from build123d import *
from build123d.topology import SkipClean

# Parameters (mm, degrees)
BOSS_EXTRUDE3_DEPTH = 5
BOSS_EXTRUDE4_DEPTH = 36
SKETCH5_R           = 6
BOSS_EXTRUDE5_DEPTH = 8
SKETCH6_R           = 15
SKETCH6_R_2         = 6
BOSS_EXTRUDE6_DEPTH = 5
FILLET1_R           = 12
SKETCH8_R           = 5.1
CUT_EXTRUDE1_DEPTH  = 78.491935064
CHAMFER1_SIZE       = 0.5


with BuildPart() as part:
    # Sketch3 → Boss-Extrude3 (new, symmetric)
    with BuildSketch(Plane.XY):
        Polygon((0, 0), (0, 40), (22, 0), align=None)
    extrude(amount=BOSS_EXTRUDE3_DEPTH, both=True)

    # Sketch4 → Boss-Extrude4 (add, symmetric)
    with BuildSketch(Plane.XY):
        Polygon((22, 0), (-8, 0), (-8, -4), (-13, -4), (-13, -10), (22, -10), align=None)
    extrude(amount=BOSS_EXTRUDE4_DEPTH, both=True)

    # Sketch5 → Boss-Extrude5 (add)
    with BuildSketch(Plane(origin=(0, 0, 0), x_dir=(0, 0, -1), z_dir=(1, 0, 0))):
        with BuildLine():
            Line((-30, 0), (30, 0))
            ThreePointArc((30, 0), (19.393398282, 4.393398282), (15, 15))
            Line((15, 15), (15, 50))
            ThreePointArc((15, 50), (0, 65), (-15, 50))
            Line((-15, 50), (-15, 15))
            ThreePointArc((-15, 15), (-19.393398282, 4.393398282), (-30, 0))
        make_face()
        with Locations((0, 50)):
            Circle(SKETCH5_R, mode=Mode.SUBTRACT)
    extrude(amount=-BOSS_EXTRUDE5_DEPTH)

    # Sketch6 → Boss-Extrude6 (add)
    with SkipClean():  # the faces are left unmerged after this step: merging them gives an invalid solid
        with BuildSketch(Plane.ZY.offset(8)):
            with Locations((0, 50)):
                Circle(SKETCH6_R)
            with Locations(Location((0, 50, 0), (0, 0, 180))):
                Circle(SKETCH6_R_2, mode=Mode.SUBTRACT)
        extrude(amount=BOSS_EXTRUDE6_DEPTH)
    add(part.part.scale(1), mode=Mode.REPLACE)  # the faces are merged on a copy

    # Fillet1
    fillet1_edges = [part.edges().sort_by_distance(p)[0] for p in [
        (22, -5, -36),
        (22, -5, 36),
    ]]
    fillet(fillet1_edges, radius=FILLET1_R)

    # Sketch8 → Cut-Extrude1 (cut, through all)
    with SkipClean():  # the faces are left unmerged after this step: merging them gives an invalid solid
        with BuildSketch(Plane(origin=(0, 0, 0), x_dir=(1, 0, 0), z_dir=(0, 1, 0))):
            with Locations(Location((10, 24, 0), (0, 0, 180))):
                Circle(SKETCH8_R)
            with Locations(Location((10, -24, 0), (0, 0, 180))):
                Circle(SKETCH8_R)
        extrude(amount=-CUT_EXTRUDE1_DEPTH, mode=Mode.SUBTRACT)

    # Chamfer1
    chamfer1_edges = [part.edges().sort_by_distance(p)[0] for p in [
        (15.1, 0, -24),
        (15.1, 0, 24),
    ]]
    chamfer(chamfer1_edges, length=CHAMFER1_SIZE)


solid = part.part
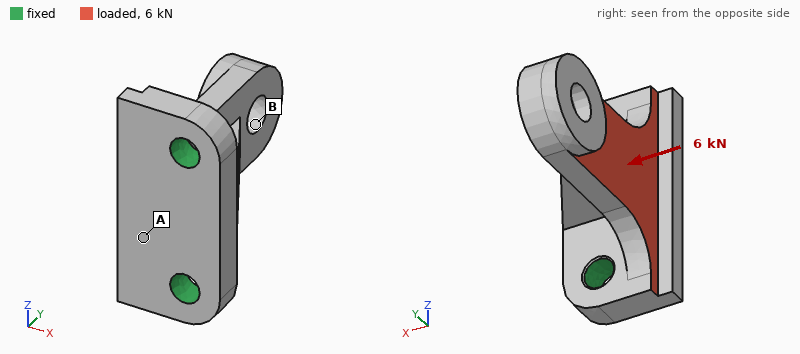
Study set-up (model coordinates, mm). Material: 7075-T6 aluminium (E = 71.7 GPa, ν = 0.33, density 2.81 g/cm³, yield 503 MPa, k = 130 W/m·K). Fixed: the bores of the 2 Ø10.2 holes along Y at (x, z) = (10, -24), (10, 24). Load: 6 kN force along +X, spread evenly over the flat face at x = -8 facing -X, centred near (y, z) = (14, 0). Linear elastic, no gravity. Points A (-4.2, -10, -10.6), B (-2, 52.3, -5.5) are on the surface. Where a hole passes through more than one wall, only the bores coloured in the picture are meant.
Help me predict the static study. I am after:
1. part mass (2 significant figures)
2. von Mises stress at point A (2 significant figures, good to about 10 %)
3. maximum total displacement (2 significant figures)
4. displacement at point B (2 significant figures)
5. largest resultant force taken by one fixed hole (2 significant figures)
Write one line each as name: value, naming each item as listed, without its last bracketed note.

part mass: 120 g
von Mises stress at point A: 23 MPa
maximum total displacement: 0.26 mm
displacement at point B: 0.21 mm
largest resultant force taken by one fixed hole: 3.1 kN
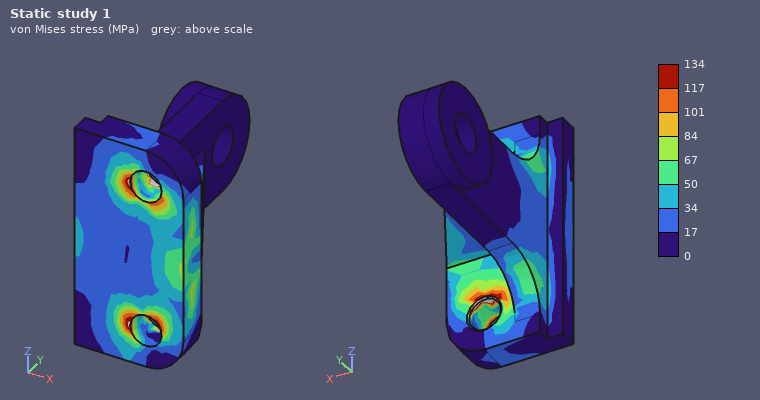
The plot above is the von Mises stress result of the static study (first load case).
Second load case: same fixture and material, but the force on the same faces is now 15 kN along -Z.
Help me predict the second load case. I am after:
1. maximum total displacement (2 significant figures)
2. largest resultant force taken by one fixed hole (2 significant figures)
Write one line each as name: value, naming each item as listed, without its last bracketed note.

maximum total displacement: 0.23 mm
largest resultant force taken by one fixed hole: 11 kN
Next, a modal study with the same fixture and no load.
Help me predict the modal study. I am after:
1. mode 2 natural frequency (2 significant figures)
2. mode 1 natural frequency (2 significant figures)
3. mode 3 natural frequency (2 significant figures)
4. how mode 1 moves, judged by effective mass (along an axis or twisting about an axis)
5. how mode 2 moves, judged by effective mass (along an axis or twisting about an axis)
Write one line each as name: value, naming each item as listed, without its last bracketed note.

mode 2 natural frequency: 4300 Hz
mode 1 natural frequency: 2500 Hz
mode 3 natural frequency: 7700 Hz
how mode 1 moves, judged by effective mass: along X
how mode 2 moves, judged by effective mass: along Z
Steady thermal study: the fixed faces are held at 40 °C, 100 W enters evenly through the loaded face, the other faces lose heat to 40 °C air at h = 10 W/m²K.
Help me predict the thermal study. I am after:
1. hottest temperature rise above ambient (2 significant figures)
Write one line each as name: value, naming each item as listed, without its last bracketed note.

hottest temperature rise above ambient: 50 K
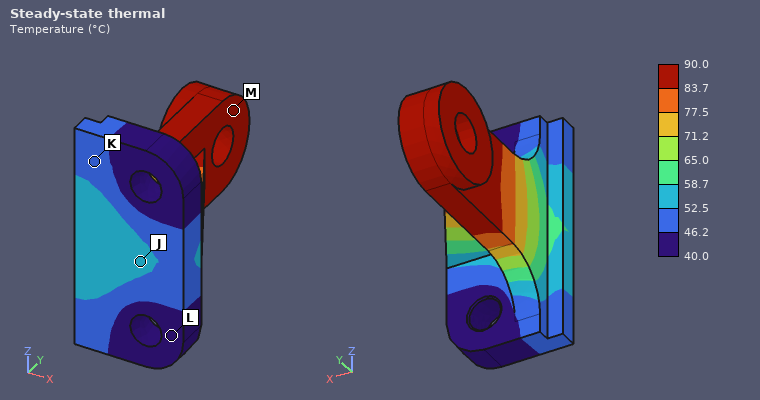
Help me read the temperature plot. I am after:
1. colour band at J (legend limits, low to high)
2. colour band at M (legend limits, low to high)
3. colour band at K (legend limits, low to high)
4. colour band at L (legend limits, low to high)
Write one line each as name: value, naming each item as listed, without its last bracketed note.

colour band at J: 52.5 to 58.7 °C
colour band at M: 83.7 to 90.0 °C
colour band at K: 46.2 to 52.5 °C
colour band at L: 40.0 to 46.2 °C
